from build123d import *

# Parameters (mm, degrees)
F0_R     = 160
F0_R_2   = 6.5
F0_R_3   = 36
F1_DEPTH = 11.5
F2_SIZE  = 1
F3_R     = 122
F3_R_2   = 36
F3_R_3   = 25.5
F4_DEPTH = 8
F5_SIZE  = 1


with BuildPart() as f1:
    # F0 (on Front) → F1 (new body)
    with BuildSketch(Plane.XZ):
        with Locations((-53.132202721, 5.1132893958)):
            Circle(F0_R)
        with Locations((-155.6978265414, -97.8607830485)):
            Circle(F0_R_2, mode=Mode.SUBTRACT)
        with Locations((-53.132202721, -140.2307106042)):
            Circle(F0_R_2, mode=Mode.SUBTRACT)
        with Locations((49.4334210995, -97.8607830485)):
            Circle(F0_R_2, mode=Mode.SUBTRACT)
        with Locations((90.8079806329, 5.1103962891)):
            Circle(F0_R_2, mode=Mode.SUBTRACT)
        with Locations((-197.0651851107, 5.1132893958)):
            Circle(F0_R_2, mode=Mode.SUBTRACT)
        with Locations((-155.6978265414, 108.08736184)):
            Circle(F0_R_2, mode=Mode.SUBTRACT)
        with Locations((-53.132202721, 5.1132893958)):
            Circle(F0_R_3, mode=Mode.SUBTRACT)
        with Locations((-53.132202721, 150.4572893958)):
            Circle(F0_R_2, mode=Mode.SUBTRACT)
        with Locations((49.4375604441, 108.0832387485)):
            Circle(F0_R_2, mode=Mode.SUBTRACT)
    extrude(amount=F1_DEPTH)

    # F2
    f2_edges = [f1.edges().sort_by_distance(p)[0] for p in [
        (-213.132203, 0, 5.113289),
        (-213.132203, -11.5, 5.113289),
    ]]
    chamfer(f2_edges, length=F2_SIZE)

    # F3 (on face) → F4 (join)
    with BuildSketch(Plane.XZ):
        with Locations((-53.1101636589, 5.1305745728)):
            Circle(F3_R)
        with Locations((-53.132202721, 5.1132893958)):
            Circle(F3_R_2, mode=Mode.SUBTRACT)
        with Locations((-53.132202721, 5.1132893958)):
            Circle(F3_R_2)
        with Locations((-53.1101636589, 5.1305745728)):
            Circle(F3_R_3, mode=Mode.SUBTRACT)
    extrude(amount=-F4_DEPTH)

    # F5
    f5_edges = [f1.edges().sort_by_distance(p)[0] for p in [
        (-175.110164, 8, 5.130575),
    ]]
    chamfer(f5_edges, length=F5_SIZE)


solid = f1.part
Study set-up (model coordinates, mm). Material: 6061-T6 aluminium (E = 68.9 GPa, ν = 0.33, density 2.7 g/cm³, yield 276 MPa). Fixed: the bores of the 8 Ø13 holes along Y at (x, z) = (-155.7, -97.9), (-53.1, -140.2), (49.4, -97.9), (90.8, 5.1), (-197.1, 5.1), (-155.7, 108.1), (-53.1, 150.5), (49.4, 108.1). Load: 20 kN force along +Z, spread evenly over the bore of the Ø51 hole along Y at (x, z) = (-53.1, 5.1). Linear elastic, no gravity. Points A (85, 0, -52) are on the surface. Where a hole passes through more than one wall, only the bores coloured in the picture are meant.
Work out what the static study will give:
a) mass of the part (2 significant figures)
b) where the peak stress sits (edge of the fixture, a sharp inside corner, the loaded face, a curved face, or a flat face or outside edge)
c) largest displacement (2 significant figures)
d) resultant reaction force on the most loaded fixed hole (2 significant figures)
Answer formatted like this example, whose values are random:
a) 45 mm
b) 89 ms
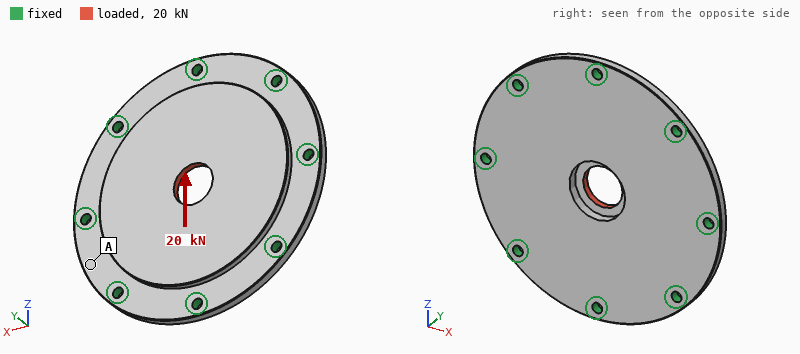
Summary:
a) 3.3 kg
b) a sharp inside corner
c) 16 µm
d) 3.9 kN
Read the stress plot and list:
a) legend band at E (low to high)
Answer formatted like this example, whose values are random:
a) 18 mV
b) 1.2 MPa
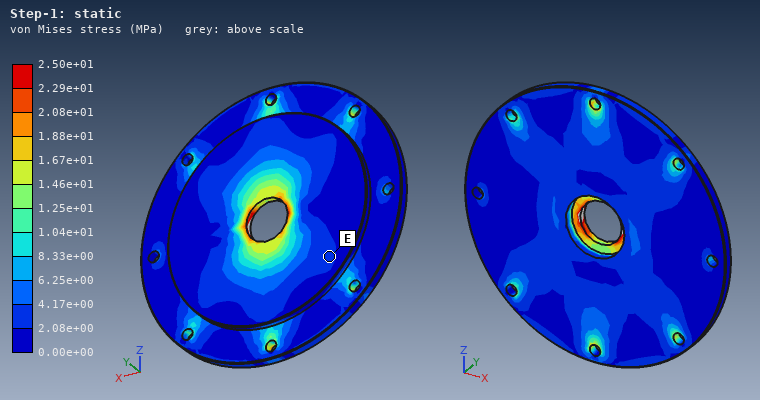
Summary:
a) 2.08e+00 to 4.17e+00 MPa
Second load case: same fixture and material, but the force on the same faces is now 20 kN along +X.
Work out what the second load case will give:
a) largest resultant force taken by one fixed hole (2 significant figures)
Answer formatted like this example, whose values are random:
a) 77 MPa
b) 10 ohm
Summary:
a) 4.0 kN
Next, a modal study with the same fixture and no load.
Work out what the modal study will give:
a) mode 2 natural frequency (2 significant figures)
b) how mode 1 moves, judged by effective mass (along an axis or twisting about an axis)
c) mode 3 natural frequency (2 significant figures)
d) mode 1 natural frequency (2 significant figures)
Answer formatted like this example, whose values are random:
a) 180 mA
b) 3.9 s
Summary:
a) 3000 Hz
b) along Y
c) 3100 Hz
d) 1500 Hz
